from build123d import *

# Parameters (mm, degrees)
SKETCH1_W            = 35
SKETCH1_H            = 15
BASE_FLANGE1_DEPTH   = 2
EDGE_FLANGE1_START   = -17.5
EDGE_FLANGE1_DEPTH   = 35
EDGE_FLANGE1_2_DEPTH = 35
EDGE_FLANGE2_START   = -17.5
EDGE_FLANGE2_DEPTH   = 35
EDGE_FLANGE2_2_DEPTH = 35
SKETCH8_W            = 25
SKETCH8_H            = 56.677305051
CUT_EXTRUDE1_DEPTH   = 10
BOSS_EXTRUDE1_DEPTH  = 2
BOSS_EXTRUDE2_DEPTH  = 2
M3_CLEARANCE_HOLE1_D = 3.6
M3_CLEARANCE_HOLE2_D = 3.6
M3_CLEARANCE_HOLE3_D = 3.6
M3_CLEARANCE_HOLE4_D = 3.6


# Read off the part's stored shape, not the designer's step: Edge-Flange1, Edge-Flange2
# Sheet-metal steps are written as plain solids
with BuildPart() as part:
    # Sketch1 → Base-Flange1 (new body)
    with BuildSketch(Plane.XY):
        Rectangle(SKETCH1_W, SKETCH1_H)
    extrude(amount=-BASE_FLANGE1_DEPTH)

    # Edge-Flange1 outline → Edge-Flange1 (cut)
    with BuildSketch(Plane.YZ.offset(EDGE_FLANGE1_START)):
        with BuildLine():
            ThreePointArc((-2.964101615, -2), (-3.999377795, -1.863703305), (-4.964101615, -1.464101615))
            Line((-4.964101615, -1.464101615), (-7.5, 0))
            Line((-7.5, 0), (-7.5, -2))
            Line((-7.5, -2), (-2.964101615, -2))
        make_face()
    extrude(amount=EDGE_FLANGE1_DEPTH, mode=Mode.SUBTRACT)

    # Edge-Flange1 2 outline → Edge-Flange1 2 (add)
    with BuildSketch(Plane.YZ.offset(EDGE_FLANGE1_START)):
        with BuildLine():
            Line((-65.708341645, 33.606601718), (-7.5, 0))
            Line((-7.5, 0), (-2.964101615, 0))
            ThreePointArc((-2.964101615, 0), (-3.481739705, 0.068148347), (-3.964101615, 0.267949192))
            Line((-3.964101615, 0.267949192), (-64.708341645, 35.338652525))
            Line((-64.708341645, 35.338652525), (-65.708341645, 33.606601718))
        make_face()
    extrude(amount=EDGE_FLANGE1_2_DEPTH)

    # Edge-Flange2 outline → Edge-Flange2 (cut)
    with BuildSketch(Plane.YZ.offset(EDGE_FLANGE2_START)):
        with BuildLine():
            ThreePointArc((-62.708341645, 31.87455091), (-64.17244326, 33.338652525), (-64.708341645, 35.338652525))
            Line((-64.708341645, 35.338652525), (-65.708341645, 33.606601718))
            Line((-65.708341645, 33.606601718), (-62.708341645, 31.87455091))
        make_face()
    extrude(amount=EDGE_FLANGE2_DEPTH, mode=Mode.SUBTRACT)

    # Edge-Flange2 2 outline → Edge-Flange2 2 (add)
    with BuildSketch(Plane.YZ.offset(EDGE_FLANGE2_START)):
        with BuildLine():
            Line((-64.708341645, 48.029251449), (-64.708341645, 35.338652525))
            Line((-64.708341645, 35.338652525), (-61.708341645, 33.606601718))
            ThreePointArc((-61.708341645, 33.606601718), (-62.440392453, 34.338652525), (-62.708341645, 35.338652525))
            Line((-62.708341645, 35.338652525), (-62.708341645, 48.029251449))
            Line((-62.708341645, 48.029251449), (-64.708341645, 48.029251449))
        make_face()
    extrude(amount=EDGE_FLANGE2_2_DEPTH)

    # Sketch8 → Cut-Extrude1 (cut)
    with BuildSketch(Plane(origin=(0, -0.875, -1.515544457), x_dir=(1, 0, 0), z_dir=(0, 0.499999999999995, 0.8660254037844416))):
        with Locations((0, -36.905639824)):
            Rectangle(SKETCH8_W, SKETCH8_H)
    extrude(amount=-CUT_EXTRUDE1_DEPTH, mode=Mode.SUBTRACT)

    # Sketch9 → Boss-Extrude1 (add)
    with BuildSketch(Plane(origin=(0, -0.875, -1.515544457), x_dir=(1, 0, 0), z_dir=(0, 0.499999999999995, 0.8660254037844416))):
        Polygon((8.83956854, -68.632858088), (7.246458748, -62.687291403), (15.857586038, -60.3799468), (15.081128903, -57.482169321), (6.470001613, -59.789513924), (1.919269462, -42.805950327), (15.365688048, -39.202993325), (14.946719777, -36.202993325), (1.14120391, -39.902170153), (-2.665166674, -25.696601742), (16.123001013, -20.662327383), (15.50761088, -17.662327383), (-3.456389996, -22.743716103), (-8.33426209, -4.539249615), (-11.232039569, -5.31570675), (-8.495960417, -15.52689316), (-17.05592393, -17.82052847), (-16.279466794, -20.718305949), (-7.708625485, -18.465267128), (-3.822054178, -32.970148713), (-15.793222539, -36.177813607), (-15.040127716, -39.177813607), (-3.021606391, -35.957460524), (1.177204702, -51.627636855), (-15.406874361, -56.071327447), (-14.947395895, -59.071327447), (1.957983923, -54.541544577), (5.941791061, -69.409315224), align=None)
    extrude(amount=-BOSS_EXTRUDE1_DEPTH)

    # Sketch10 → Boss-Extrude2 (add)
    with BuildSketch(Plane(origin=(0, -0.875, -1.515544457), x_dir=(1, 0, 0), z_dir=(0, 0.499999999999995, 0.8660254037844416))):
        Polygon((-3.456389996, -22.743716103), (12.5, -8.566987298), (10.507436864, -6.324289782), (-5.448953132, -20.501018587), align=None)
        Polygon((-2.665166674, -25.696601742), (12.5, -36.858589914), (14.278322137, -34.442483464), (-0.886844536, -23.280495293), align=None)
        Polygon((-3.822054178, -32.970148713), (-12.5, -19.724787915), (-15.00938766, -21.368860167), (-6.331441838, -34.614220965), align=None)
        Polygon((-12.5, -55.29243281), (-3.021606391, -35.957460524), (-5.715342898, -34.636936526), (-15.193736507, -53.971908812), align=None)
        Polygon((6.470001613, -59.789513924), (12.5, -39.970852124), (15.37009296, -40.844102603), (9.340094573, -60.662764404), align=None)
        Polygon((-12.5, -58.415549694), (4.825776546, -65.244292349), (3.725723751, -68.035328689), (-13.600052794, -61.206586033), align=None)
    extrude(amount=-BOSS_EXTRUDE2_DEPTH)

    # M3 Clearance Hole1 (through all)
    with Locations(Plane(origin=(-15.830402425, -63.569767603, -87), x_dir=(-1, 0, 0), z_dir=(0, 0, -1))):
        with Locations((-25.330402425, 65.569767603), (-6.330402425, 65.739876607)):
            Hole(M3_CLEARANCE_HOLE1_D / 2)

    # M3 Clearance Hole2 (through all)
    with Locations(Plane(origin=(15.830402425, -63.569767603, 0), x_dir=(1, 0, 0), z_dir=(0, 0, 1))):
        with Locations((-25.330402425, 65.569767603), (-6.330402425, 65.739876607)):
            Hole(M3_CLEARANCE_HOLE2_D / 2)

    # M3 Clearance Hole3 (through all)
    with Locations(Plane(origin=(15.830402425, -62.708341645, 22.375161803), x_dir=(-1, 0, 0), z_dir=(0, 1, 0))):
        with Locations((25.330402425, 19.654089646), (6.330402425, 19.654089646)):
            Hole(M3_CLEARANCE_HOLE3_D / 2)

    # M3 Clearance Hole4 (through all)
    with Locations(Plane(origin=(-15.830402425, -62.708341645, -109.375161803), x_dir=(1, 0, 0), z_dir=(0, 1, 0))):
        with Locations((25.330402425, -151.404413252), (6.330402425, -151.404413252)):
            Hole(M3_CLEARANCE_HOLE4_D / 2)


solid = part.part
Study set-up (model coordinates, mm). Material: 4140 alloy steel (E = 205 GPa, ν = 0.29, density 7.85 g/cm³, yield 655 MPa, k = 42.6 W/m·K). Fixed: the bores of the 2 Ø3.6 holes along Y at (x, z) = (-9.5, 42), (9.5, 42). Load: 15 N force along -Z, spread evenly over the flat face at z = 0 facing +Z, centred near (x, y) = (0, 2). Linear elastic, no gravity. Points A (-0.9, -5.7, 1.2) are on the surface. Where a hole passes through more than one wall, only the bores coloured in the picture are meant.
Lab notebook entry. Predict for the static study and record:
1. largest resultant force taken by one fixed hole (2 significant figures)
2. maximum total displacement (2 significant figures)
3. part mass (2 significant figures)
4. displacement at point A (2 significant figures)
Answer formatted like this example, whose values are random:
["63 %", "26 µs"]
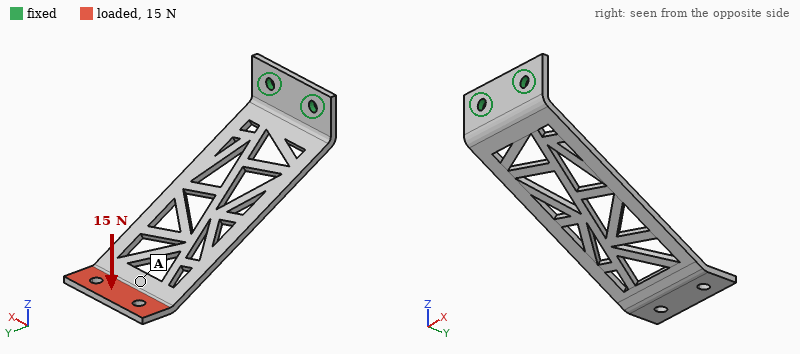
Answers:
["9.3 N", "0.95 mm", "39 g", "0.73 mm"]
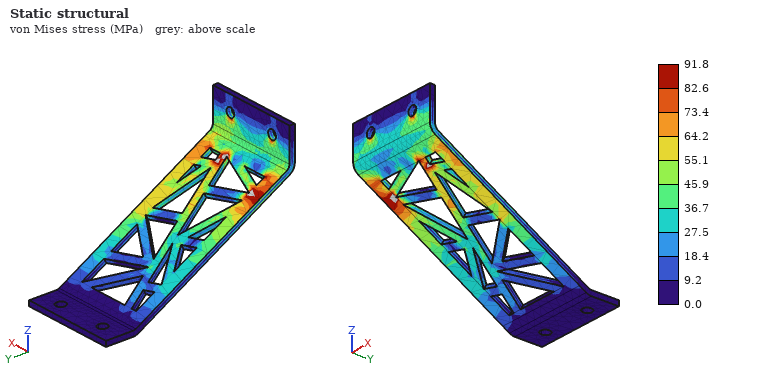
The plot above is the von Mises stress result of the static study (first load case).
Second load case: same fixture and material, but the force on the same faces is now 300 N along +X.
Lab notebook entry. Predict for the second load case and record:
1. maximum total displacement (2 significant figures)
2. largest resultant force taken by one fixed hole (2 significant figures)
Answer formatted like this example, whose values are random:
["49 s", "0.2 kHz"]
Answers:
["0.80 mm", "1.1 kN"]
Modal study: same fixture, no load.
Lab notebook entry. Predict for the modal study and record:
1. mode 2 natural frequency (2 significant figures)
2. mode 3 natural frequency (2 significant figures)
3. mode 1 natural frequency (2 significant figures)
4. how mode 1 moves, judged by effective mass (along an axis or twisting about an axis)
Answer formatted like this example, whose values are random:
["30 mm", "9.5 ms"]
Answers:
["840 Hz", "1200 Hz", "190 Hz", "along Z"]
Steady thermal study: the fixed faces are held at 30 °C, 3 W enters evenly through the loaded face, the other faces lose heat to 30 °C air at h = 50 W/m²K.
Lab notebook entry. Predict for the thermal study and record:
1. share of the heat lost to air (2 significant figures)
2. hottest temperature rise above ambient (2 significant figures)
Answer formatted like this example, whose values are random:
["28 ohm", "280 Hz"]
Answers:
["96 %", "34 K"]
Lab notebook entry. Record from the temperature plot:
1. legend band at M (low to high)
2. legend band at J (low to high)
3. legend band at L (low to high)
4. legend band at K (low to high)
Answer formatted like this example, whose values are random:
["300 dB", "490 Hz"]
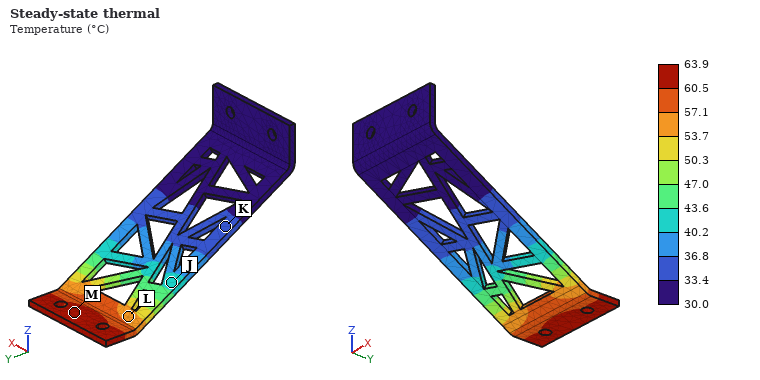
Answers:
["60.5 to 63.9 °C", "40.2 to 43.6 °C", "53.7 to 57.1 °C", "33.4 to 36.8 °C"]
